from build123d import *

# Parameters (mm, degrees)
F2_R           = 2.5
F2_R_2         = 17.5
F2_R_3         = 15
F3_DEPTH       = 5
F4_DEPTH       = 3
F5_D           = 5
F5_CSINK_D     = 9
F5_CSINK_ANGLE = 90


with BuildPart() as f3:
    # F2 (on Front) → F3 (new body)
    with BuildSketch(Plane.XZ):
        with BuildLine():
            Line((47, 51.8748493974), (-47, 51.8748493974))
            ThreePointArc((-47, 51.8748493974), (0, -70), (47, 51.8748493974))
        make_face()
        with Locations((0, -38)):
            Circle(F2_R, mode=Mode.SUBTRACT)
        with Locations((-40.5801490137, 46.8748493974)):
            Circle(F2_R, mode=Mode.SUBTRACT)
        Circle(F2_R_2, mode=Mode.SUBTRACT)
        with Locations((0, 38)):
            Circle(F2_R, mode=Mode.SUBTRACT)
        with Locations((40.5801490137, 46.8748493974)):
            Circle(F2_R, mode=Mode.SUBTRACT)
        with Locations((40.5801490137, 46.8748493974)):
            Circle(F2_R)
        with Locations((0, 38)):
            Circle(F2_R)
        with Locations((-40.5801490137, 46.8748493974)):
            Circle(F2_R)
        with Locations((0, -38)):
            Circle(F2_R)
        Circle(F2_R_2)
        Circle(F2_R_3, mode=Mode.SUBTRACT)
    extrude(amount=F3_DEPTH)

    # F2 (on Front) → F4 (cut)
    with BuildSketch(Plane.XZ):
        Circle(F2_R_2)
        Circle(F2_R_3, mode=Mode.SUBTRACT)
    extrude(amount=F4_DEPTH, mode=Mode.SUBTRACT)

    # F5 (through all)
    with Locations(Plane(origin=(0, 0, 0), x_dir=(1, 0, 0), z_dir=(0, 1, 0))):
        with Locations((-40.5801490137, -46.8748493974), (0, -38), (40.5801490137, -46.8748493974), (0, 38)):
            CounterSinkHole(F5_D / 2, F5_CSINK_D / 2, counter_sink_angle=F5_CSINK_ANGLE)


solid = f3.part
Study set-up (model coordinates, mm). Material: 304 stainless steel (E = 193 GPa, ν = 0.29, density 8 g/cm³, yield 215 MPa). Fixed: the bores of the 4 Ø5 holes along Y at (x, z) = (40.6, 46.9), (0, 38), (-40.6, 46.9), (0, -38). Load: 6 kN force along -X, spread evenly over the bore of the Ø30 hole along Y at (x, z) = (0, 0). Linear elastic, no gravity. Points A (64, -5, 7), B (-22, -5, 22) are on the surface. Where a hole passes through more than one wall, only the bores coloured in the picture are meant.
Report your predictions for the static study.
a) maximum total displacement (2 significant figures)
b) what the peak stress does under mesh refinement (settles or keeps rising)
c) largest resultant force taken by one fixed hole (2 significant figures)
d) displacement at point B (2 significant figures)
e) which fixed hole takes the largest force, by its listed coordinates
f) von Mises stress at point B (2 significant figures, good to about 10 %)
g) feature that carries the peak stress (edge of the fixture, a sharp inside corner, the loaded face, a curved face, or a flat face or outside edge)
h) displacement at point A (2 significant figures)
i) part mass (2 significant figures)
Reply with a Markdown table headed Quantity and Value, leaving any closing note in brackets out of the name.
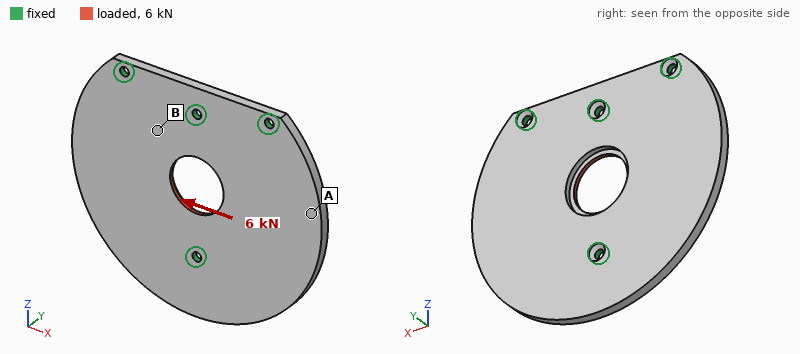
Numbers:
| Quantity | Value |
|---|---|
| maximum total displacement | 15 µm |
| what the peak stress does under mesh refinement | keeps rising |
| largest resultant force taken by one fixed hole | 2.9 kN |
| displacement at point B | 3.6 µm |
| which fixed hole takes the largest force, by its listed coordinates | (0, -38) |
| von Mises stress at point B | 16 MPa |
| feature that carries the peak stress | edge of the fixture |
| displacement at point A | 11 µm |
| part mass | 530 g |
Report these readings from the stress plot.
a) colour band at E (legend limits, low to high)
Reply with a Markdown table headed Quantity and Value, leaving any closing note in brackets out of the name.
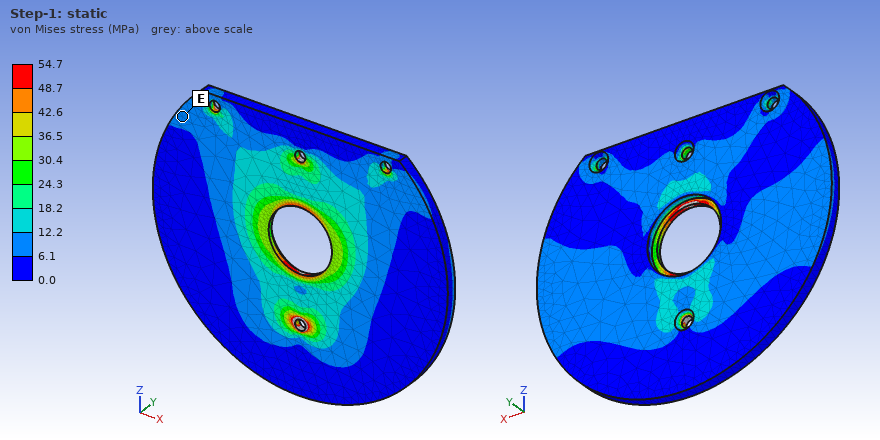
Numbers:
| Quantity | Value |
|---|---|
| colour band at E | 6.1 to 12.2 MPa |
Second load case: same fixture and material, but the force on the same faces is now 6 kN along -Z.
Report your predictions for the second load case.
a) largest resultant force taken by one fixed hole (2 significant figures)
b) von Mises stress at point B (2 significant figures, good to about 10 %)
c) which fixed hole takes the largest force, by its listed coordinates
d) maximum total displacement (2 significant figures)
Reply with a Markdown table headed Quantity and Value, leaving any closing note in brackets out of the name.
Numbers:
| Quantity | Value |
|---|---|
| largest resultant force taken by one fixed hole | 2.2 kN |
| von Mises stress at point B | 11 MPa |
| which fixed hole takes the largest force, by its listed coordinates | (0, -38) |
| maximum total displacement | 4.1 µm |
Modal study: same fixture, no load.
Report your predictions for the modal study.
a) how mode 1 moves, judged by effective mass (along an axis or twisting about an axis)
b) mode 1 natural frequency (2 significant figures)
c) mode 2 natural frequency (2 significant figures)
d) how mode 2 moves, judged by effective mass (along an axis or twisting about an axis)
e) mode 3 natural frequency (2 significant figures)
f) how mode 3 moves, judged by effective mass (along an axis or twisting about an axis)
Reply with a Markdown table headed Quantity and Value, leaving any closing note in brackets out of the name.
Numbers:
| Quantity | Value |
|---|---|
| how mode 1 moves, judged by effective mass | twisting about Z |
| mode 1 natural frequency | 1000 Hz |
| mode 2 natural frequency | 1300 Hz |
| how mode 2 moves, judged by effective mass | along Y |
| mode 3 natural frequency | 2500 Hz |
| how mode 3 moves, judged by effective mass | twisting about X |
